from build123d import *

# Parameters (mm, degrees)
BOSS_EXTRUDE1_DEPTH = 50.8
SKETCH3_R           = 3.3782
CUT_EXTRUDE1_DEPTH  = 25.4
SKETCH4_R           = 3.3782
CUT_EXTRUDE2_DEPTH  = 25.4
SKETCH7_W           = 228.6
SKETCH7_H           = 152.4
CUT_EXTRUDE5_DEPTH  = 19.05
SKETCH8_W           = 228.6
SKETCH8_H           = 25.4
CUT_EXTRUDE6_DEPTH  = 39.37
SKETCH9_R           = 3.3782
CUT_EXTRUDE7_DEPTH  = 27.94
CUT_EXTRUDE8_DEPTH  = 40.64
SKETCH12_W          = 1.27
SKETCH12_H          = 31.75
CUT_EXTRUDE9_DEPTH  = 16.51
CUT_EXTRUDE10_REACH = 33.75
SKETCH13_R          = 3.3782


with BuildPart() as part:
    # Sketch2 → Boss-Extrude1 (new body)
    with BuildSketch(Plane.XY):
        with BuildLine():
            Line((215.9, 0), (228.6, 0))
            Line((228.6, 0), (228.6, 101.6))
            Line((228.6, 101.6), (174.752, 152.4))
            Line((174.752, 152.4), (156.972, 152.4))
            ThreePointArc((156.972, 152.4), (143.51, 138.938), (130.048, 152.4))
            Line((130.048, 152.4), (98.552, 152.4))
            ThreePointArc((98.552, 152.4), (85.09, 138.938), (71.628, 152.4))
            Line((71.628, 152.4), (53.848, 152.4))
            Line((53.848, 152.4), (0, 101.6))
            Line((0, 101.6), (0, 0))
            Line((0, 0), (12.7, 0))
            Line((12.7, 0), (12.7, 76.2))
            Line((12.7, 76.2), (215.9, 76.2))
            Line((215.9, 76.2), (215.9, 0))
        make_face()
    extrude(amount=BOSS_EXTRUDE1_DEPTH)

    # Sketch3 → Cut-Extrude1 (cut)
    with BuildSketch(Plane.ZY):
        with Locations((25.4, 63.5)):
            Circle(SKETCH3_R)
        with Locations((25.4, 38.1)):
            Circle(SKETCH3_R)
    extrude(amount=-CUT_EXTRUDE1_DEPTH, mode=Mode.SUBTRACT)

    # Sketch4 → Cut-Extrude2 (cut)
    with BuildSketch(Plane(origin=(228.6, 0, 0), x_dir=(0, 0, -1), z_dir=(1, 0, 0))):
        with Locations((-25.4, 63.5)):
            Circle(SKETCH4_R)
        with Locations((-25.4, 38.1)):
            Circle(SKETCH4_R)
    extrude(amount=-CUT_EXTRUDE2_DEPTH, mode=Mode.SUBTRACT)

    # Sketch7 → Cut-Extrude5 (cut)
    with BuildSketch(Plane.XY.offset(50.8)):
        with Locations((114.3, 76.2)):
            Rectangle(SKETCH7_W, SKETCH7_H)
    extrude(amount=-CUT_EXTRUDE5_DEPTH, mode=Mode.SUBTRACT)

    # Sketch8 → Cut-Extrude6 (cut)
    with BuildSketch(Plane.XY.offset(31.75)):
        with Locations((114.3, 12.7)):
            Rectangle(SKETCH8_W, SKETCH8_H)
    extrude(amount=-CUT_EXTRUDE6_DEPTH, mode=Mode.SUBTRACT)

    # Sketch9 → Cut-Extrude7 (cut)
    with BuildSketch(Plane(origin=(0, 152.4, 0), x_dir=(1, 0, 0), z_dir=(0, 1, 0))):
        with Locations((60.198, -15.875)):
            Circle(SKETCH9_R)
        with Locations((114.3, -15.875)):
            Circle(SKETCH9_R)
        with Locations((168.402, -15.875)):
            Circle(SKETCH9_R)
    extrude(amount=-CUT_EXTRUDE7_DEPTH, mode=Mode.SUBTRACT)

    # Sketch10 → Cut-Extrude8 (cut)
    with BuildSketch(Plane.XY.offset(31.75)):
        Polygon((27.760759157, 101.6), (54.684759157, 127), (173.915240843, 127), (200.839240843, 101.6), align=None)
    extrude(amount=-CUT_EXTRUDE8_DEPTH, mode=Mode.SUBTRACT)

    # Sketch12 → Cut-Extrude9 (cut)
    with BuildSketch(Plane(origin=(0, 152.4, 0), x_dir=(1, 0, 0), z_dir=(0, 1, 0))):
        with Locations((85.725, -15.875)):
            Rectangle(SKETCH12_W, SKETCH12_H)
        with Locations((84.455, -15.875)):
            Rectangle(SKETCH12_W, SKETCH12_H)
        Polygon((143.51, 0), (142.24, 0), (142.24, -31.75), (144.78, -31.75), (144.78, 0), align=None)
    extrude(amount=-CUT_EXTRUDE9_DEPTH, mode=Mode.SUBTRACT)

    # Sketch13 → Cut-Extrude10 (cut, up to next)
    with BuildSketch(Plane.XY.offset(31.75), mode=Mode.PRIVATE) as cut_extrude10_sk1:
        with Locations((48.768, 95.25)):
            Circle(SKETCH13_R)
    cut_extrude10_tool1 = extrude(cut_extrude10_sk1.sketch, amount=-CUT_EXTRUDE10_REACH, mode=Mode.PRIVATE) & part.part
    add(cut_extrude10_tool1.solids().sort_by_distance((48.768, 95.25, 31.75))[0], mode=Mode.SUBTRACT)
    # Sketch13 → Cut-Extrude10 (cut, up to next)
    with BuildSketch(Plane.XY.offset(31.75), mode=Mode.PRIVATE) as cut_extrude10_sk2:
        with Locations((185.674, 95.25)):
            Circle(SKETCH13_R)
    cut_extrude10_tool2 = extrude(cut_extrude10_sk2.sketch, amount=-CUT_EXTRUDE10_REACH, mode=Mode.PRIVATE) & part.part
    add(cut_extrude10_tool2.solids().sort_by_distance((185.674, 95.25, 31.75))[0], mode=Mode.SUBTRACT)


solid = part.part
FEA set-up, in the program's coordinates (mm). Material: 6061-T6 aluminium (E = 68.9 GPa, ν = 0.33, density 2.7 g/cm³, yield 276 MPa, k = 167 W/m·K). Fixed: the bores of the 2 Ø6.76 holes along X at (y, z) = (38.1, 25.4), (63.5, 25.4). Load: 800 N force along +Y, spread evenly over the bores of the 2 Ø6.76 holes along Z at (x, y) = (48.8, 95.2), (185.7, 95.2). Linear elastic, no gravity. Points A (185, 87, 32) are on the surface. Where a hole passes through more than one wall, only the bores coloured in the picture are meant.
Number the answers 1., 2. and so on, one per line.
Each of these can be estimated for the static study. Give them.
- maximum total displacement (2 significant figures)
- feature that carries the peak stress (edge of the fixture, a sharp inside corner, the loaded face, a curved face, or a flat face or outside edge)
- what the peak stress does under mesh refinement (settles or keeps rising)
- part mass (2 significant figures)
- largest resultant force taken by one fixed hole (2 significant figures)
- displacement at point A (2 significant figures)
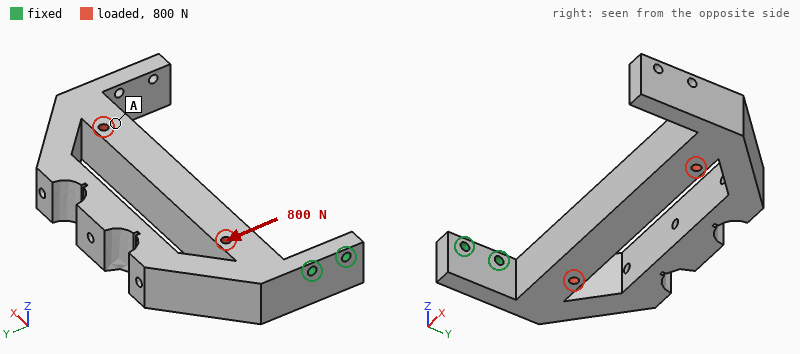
1. 1.3 mm
2. edge of the fixture
3. keeps rising
4. 980 g
5. 1.3 kN
6. 0.99 mm
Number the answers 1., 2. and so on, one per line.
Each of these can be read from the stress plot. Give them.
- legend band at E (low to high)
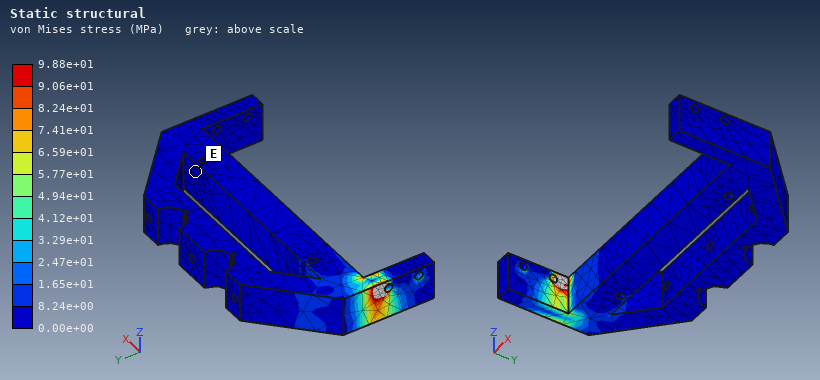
1. 0.00e+00 to 8.24e+00 MPa
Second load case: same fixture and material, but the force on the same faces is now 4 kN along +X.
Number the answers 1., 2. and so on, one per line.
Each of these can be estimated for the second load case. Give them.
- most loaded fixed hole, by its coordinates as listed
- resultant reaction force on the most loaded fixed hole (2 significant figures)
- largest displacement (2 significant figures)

1. (63.5, 25.4)
2. 5.4 kN
3. 1.3 mm
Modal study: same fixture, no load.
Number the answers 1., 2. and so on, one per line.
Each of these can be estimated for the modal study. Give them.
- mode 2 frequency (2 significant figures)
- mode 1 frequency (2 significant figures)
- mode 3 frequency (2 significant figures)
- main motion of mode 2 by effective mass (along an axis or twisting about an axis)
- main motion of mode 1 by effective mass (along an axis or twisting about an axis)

1. 170 Hz
2. 150 Hz
3. 850 Hz
4. along Z
5. along Y
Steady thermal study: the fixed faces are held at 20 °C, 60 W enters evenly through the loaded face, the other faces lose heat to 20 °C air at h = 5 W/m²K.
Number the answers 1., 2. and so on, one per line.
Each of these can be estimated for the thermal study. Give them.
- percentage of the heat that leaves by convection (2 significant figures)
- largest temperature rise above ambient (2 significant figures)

1. 16 %
2. 46 K
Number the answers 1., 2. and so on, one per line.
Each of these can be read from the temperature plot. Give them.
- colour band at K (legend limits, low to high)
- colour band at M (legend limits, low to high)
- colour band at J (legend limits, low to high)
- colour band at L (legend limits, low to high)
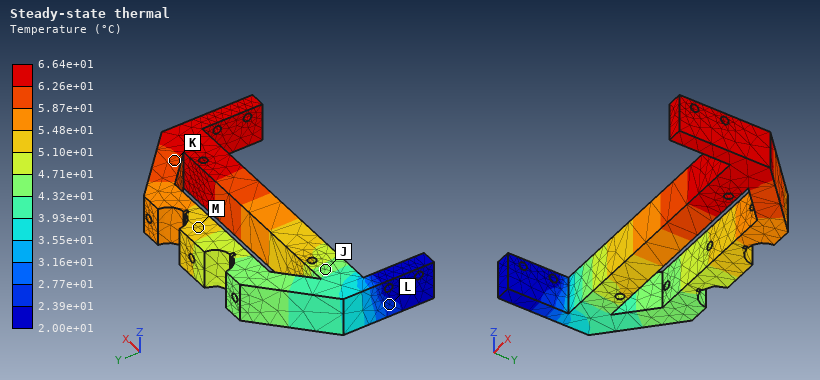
1. 5.87e+01 to 6.26e+01 °C
2. 5.10e+01 to 5.48e+01 °C
3. 4.32e+01 to 4.71e+01 °C
4. 2.39e+01 to 2.77e+01 °C
